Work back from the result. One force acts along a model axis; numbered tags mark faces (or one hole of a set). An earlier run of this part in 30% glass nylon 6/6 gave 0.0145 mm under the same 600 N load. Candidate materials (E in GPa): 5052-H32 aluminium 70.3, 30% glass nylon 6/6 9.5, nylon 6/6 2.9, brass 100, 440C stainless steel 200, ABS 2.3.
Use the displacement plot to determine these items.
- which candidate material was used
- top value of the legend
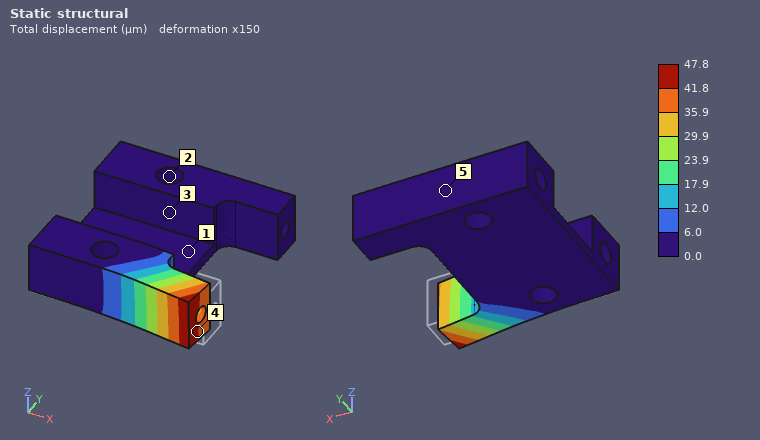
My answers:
nylon 6/6
47.8 µm
